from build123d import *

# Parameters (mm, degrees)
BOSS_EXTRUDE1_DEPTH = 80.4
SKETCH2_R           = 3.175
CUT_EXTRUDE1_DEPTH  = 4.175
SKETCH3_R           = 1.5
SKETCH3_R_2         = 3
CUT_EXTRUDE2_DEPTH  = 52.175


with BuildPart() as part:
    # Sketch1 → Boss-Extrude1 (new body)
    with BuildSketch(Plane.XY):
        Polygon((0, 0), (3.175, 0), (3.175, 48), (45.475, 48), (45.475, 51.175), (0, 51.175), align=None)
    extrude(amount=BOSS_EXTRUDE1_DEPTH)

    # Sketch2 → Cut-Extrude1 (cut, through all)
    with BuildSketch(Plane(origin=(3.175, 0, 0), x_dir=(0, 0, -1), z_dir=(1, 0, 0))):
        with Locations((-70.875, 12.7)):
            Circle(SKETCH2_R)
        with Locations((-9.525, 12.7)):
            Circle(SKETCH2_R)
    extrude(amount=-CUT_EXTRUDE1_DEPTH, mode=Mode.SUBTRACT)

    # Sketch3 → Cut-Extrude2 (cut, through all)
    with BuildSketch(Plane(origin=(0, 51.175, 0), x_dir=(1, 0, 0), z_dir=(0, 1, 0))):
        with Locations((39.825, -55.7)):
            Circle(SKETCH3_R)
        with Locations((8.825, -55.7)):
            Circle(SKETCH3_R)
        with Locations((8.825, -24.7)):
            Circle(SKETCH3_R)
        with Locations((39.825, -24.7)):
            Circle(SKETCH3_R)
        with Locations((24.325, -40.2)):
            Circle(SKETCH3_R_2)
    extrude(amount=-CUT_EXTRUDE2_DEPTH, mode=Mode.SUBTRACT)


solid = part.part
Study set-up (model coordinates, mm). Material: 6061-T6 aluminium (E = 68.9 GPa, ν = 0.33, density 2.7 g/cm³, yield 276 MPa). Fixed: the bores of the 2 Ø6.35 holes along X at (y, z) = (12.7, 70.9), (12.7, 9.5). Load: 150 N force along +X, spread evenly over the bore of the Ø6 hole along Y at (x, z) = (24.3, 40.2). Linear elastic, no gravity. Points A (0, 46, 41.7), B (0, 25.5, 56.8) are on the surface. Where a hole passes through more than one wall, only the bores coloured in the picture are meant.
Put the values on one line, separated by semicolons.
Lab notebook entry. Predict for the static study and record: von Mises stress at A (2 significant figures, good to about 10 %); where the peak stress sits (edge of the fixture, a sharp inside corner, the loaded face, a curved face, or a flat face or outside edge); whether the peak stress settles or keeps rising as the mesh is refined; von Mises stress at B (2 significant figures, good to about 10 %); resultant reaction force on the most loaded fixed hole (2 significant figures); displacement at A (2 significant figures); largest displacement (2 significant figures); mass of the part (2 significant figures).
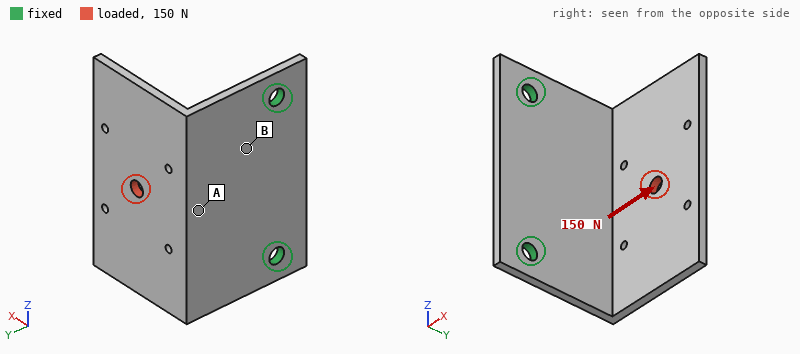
6.5 MPa; edge of the fixture; keeps rising; 22 MPa; 75 N; 0.16 mm; 0.38 mm; 63 g
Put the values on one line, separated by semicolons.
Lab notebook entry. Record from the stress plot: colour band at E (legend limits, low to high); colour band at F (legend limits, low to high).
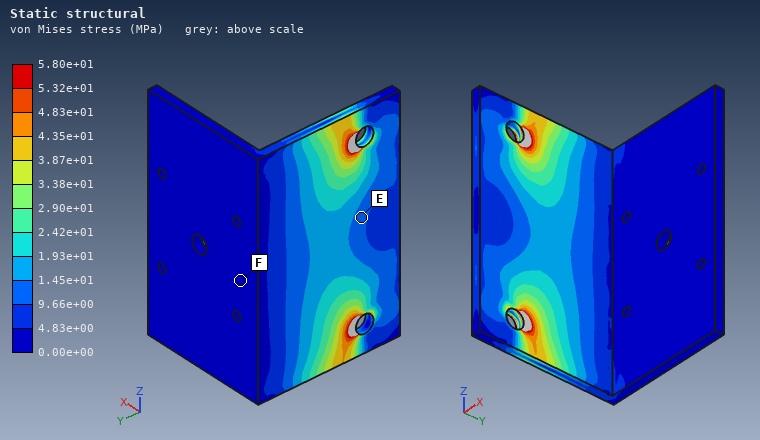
9.66e+00 to 1.45e+01 MPa; 0.00e+00 to 4.83e+00 MPa
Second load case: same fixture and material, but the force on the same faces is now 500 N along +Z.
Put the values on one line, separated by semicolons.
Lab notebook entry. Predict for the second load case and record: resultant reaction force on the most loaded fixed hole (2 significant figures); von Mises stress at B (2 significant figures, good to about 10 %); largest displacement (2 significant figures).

420 N; 27 MPa; 0.41 mm
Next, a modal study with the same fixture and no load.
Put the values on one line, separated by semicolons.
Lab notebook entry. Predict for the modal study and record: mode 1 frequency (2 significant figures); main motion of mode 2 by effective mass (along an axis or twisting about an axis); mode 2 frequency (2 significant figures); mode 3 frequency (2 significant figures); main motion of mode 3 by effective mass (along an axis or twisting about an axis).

530 Hz; along Z; 1000 Hz; 1400 Hz; along X
